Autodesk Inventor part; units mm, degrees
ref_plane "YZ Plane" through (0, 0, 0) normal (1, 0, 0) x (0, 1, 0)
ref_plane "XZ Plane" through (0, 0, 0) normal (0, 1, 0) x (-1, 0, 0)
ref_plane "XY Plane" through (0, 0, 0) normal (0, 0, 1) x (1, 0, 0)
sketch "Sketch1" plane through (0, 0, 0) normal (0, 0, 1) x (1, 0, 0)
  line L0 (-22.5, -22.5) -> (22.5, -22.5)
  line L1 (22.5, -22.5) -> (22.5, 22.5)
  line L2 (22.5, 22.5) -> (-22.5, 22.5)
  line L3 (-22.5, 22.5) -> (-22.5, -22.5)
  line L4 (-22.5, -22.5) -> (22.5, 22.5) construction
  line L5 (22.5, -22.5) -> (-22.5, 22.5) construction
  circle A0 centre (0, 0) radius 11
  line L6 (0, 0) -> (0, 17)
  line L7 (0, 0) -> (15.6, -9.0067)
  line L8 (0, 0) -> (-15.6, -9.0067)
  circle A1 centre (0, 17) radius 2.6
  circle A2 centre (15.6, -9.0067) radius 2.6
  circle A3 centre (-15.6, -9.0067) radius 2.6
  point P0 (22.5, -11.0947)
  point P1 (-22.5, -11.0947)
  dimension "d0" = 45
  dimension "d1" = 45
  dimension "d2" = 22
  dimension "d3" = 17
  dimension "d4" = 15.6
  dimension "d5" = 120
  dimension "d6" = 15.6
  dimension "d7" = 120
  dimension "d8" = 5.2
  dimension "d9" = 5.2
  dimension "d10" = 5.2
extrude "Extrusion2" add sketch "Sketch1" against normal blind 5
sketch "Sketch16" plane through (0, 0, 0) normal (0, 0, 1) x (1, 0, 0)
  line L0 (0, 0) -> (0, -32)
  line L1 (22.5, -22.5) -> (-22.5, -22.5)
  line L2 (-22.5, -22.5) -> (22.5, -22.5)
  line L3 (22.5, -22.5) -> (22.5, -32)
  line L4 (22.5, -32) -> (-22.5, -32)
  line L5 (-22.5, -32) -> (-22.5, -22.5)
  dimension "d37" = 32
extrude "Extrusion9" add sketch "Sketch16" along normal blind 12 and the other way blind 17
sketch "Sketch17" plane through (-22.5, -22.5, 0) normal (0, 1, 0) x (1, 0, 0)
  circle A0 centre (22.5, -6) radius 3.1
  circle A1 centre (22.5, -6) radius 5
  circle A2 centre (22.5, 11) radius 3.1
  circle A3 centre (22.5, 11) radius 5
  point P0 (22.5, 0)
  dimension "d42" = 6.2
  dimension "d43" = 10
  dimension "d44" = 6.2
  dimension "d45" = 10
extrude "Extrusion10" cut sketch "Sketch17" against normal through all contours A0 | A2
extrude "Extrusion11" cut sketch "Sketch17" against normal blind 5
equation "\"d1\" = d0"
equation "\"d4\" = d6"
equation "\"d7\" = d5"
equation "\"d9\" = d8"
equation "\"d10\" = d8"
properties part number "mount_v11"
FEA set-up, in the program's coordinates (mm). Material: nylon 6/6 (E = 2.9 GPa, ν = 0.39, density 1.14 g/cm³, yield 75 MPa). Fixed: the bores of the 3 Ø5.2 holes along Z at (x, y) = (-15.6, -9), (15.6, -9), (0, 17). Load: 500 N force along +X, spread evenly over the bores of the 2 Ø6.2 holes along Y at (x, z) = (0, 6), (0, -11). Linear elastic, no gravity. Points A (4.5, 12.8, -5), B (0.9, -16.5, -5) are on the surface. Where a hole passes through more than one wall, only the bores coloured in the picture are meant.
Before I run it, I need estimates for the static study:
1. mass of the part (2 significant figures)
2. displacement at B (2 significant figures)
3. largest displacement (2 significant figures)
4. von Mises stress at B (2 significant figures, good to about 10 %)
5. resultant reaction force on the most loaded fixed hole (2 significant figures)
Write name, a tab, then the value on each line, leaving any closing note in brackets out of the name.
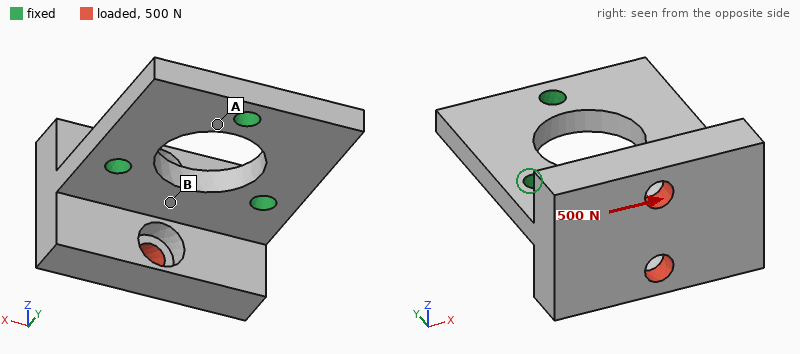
mass of the part	22 g
displacement at B	23 µm
largest displacement	69 µm
von Mises stress at B	4.8 MPa
resultant reaction force on the most loaded fixed hole	380 N
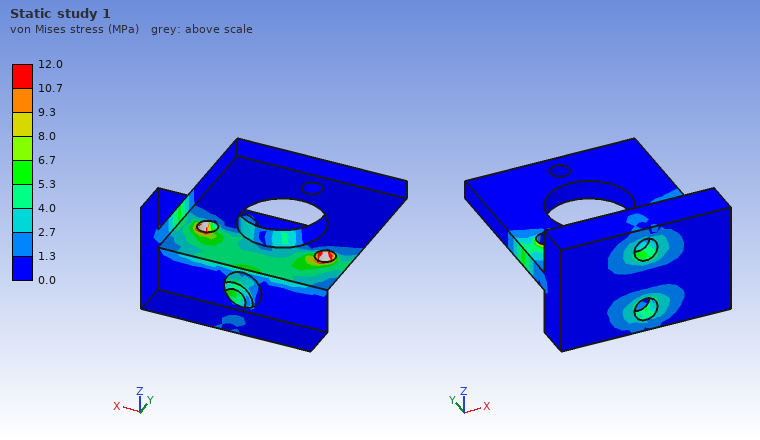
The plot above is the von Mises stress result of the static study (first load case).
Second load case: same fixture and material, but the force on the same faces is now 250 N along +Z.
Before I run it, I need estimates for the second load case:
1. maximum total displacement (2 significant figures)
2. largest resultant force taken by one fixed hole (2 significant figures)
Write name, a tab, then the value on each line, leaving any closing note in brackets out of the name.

maximum total displacement	0.87 mm
largest resultant force taken by one fixed hole	130 N
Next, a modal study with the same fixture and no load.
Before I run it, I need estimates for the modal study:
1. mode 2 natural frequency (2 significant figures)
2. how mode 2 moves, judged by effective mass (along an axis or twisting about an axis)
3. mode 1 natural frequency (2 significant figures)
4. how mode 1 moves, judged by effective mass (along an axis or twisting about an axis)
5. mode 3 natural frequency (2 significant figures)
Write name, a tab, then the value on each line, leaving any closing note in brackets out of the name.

mode 2 natural frequency	2200 Hz
how mode 2 moves, judged by effective mass	twisting about Y
mode 1 natural frequency	900 Hz
how mode 1 moves, judged by effective mass	along Z
mode 3 natural frequency	3600 Hz
